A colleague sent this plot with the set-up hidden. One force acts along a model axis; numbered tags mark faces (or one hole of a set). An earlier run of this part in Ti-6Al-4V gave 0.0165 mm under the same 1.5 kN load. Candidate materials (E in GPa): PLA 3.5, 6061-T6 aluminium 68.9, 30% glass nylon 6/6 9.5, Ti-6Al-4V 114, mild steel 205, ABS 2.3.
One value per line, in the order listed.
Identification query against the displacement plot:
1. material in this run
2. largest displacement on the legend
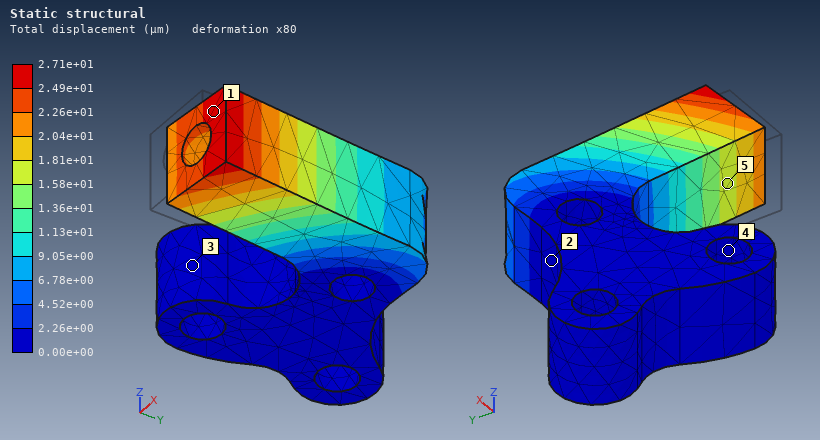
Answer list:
6061-T6 aluminium
2.71e+01 µm
